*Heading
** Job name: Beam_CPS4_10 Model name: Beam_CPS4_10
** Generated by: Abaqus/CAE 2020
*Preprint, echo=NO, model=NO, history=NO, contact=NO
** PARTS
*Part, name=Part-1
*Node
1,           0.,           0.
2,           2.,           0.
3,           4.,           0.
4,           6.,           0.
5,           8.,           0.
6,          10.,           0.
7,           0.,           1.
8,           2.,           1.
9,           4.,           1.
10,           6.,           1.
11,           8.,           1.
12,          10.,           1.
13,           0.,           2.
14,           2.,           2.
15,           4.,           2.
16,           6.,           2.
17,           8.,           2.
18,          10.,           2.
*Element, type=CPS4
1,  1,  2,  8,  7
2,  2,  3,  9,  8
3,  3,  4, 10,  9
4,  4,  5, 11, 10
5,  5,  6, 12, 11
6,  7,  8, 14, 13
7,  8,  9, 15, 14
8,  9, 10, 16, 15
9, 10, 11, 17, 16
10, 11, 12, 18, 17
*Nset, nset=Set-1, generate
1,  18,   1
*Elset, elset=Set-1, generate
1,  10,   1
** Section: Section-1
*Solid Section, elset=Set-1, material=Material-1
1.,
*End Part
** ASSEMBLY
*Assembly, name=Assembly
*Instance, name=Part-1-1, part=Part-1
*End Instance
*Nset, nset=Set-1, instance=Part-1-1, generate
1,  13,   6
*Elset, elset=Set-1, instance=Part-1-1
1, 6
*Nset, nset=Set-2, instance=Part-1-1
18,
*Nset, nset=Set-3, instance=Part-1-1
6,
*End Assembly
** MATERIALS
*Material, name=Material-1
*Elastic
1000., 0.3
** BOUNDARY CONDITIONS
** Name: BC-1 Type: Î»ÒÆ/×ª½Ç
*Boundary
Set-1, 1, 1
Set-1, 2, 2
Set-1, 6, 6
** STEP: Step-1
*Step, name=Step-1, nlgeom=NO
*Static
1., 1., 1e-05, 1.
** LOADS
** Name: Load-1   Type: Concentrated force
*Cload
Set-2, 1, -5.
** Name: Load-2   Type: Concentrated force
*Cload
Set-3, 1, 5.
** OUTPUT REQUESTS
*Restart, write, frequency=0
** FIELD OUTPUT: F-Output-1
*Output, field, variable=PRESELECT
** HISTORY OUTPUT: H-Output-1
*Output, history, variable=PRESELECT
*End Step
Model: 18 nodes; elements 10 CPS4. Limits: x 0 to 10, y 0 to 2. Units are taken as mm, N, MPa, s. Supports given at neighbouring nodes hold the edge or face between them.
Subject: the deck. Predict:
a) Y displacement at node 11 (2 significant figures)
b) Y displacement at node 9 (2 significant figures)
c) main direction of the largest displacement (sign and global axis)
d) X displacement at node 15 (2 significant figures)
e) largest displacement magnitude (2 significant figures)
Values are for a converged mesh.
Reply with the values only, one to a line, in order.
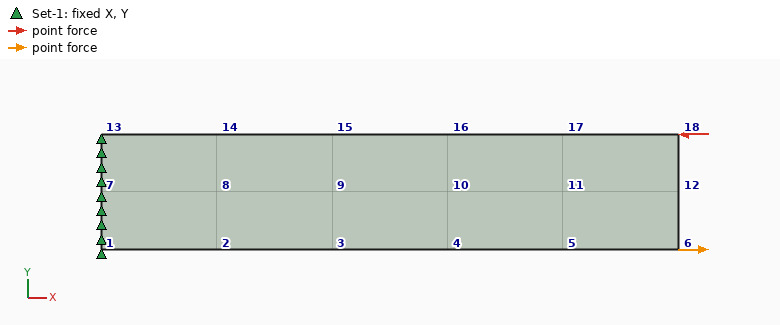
0.47 mm
0.12 mm
+Y
-0.059 mm
0.77 mm
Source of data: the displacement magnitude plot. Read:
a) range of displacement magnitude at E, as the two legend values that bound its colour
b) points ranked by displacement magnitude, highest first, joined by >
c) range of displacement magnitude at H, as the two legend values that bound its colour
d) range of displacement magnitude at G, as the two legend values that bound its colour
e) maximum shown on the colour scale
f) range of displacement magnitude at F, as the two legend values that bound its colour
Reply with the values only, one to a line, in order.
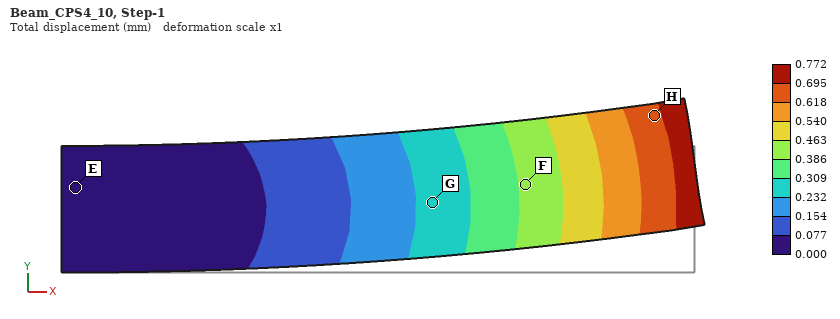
0.000 to 0.077 mm
H > F > G > E
0.618 to 0.695 mm
0.232 to 0.309 mm
0.772 mm
0.386 to 0.463 mm
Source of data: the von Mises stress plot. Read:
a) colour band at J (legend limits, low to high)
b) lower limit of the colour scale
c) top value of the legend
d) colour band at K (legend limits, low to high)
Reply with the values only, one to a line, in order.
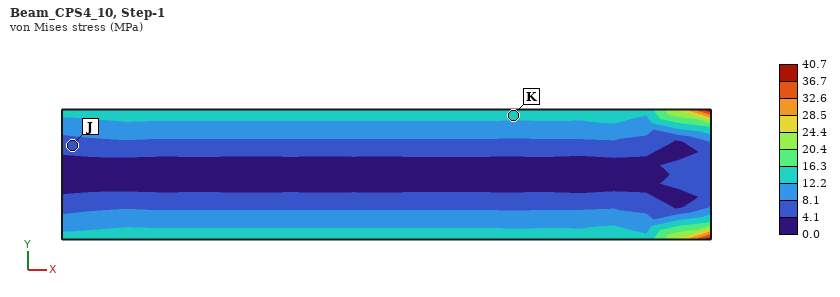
4.1 to 8.1 MPa
0.0 MPa
40.7 MPa
12.2 to 16.3 MPa
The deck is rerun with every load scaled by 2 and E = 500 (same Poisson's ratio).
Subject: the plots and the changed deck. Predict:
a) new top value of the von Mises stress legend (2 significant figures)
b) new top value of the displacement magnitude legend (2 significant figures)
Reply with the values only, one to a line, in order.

81 MPa
3.1 mm
